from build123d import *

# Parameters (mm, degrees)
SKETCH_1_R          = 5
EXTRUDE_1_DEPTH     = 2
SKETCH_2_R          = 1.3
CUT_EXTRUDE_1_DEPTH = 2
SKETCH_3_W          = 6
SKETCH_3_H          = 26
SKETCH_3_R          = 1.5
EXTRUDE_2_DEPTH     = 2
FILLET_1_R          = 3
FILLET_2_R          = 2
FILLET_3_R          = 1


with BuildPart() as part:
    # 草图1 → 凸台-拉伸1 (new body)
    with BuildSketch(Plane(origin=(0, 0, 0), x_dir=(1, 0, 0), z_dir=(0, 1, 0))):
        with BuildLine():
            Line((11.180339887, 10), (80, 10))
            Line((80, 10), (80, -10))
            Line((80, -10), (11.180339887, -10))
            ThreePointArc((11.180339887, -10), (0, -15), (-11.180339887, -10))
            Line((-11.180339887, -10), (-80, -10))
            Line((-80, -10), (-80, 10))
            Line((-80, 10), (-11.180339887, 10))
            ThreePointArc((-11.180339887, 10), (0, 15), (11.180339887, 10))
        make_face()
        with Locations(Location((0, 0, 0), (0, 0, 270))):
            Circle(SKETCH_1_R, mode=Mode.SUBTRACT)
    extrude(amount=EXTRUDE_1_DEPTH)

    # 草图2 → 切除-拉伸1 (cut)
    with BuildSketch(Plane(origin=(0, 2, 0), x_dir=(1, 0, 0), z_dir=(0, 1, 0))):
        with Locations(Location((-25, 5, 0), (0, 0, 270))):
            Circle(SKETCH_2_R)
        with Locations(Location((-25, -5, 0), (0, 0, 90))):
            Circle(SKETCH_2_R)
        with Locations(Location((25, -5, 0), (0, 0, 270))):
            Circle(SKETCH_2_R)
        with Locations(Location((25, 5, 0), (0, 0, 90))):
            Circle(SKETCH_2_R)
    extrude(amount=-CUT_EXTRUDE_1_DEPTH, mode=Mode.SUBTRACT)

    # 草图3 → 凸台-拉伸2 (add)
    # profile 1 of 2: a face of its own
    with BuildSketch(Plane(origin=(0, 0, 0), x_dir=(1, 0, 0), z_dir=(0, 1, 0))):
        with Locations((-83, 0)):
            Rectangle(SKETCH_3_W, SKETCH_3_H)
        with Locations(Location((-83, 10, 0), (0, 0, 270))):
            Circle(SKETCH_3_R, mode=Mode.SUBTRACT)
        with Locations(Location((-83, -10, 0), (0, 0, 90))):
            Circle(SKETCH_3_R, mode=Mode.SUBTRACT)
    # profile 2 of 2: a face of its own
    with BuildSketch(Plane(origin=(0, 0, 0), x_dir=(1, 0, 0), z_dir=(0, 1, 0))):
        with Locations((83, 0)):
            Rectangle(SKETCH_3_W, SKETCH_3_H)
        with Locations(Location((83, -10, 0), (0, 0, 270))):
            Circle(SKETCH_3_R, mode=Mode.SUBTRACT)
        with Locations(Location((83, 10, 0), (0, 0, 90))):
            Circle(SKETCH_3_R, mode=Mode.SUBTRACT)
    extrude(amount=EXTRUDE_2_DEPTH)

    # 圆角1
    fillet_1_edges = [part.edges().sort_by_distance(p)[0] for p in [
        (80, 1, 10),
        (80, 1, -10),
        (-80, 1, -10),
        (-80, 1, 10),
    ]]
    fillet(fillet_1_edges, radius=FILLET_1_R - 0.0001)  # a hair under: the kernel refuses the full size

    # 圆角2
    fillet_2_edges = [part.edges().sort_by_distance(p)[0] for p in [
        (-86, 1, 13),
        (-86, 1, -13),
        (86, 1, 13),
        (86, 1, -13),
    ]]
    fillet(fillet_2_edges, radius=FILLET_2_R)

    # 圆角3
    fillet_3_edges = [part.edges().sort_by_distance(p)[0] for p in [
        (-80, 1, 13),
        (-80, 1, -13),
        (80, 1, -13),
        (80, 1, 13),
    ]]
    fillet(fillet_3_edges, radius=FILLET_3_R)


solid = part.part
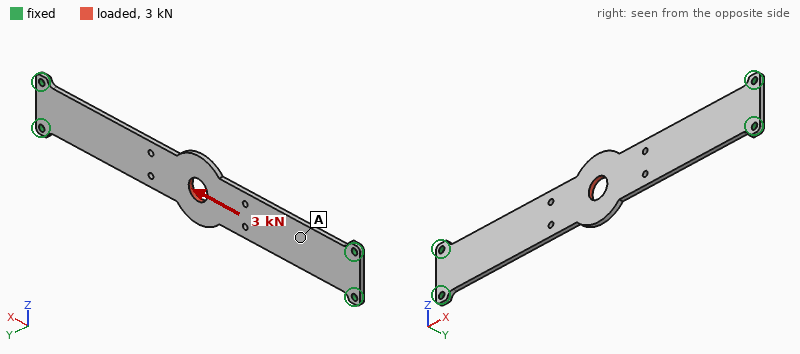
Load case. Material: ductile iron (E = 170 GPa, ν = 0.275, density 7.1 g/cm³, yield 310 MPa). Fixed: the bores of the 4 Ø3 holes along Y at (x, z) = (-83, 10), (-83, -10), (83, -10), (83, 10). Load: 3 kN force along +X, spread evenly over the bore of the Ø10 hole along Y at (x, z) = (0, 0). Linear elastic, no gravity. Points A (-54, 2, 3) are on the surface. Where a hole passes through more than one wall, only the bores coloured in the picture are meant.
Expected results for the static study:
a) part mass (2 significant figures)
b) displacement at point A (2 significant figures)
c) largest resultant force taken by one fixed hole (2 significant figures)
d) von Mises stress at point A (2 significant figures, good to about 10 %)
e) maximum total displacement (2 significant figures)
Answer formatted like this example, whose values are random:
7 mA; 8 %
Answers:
50 g; 7.6 µm; 790 N; 38 MPa; 20 µm
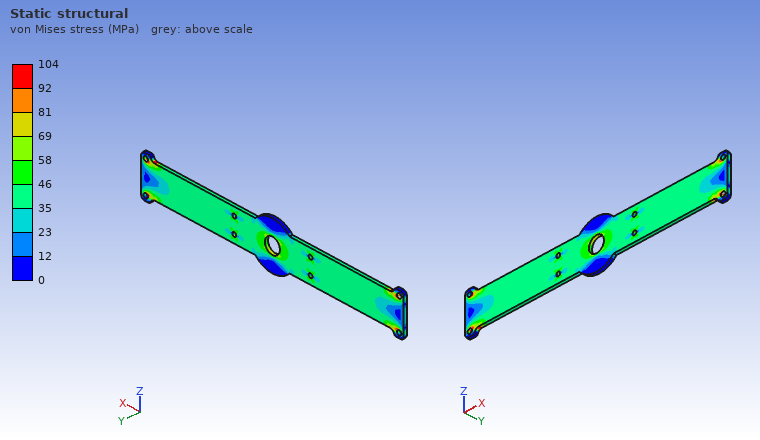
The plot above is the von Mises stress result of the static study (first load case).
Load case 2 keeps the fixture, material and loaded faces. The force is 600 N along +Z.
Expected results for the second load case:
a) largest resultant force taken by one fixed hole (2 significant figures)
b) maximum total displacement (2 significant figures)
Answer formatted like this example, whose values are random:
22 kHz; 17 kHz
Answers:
630 N; 62 µm
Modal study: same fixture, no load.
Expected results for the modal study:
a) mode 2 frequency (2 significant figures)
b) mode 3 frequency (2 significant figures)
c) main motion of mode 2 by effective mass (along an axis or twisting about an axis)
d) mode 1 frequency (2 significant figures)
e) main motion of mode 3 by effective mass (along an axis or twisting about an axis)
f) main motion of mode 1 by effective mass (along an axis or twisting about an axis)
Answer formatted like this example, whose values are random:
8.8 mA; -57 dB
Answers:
990 Hz; 1600 Hz; twisting about Z; 350 Hz; twisting about X; along Y
